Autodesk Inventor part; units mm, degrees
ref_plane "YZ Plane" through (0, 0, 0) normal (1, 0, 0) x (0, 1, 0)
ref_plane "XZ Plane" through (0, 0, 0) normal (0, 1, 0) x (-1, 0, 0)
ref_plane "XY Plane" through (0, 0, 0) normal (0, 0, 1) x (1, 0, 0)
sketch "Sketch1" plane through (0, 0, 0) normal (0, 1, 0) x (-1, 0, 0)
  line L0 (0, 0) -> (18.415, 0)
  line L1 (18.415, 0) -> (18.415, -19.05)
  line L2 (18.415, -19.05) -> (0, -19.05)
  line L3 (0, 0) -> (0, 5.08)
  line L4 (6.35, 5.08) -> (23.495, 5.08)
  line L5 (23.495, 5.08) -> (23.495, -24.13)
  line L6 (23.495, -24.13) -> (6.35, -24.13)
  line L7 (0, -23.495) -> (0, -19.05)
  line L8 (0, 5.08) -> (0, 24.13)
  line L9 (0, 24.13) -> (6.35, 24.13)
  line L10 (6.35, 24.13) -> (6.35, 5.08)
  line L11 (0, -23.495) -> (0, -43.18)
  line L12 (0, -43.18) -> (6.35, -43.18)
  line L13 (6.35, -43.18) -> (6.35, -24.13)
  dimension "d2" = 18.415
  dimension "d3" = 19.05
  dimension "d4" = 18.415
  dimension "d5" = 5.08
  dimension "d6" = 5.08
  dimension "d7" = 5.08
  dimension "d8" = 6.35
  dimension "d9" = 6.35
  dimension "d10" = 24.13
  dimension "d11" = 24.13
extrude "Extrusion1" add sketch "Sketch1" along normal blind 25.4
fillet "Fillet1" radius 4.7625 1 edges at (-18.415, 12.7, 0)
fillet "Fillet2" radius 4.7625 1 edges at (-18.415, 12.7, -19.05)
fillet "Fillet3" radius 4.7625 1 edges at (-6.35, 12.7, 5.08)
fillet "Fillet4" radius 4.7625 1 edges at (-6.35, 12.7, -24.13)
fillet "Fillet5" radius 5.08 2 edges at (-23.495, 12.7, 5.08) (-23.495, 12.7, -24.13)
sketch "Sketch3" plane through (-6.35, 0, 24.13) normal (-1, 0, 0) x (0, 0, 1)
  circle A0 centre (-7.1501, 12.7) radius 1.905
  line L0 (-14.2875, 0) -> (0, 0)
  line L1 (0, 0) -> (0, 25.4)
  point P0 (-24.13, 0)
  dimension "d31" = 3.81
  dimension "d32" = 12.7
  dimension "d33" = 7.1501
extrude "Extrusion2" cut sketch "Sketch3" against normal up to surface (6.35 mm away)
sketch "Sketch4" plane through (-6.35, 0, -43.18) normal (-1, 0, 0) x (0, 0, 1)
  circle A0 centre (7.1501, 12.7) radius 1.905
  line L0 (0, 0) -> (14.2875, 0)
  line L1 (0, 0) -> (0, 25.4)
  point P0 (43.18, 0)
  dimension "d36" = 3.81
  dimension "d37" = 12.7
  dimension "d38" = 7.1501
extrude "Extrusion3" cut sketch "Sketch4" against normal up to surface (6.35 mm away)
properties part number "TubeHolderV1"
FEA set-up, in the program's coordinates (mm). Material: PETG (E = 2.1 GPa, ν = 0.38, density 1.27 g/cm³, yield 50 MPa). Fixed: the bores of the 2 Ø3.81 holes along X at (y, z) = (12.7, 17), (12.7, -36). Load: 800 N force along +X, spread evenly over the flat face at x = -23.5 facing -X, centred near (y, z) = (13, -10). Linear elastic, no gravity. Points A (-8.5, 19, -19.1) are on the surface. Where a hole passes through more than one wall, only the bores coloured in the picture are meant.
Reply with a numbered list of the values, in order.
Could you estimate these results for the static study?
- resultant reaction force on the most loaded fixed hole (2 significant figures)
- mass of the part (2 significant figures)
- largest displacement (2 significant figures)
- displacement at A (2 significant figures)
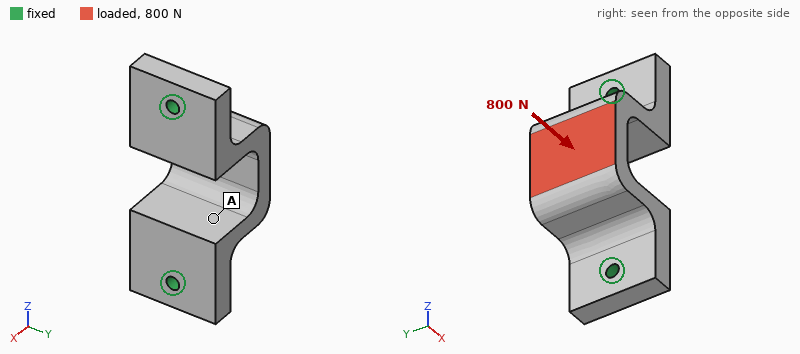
1. 500 N
2. 19 g
3. 0.26 mm
4. 0.20 mm
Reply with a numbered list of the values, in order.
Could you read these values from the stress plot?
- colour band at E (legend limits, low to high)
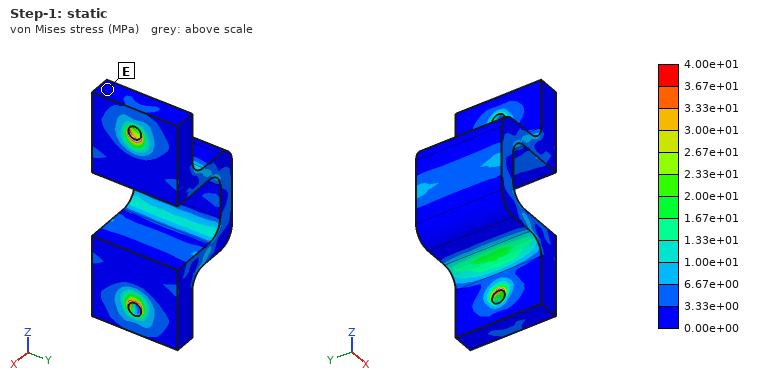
1. 0.00e+00 to 3.33e+00 MPa
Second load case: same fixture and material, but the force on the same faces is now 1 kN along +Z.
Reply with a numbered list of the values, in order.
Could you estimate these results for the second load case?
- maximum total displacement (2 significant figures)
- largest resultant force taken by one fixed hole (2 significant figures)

1. 0.39 mm
2. 660 N
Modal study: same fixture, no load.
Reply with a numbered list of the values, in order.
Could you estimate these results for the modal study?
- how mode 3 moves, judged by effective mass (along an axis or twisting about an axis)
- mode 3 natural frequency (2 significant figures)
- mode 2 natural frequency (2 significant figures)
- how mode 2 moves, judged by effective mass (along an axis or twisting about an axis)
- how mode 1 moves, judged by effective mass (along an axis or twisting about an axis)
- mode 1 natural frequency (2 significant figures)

1. along Z
2. 2900 Hz
3. 2700 Hz
4. along X
5. along Y
6. 1300 Hz
